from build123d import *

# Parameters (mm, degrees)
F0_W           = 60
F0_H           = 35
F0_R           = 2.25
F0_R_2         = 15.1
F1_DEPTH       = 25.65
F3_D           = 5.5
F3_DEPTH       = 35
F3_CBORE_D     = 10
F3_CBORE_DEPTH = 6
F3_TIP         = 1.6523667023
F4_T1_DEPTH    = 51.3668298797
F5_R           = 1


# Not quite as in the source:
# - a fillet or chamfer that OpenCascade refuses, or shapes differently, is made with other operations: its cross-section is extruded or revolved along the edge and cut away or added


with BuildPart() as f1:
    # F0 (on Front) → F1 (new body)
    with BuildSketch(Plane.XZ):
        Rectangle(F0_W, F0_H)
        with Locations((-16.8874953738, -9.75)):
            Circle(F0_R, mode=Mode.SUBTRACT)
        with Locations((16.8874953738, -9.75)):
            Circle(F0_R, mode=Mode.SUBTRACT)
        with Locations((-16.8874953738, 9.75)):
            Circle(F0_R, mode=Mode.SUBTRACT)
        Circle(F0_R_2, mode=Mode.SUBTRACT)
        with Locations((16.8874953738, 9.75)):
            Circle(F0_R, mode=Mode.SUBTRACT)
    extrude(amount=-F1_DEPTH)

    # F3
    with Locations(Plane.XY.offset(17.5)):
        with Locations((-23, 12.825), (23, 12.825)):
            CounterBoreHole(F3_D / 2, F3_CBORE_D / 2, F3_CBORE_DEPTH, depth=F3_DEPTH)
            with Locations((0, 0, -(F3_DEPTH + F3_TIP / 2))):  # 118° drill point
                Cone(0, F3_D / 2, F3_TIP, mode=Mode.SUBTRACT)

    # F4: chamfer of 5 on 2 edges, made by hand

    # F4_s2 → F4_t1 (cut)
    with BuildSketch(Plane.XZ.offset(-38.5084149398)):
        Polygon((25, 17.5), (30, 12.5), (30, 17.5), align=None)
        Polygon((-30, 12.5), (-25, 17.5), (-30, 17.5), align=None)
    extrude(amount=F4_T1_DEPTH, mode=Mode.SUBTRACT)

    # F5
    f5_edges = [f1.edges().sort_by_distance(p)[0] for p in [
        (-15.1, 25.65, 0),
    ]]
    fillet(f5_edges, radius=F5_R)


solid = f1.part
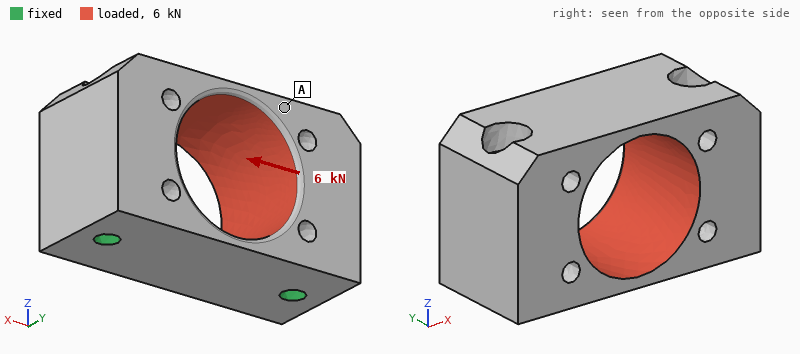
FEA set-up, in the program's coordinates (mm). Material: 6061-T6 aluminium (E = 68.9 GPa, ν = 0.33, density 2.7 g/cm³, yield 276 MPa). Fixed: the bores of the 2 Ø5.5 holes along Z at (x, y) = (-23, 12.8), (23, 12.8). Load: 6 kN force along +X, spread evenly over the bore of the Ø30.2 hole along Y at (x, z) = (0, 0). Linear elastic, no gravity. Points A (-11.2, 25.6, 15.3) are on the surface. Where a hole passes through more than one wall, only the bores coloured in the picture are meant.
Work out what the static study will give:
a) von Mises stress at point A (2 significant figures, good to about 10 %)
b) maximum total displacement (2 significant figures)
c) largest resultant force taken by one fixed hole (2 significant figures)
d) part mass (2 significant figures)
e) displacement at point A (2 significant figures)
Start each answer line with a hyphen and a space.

- 4.1 MPa
- 4.7 µm
- 3.0 kN
- 84 g
- 3.9 µm
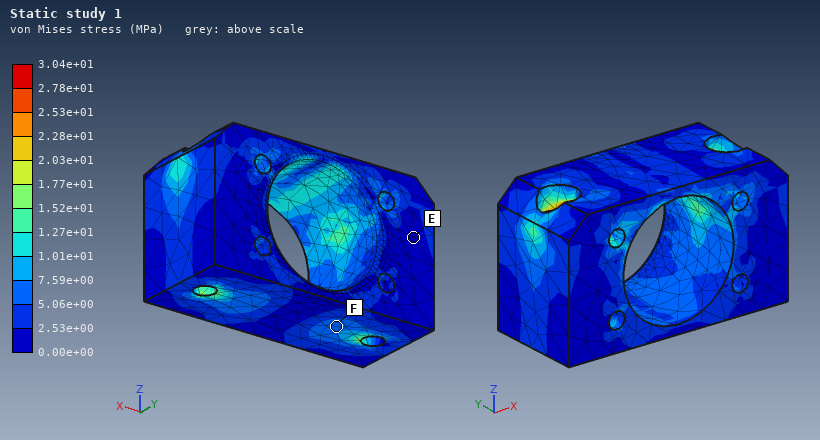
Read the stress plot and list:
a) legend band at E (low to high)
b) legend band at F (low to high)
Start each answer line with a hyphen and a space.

- 0.00e+00 to 2.53e+00 MPa
- 5.06e+00 to 7.59e+00 MPa
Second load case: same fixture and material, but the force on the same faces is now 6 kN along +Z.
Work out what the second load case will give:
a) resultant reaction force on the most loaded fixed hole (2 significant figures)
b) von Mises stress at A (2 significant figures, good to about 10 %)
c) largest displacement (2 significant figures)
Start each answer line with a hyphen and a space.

- 3.0 kN
- 3.5 MPa
- 12 µm
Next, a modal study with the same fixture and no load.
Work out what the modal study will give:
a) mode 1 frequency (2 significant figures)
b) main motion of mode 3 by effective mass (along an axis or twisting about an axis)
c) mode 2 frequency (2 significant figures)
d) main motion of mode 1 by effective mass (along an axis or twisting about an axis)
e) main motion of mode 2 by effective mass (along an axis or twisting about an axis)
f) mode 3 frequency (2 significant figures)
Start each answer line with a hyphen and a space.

- 21 kHz
- twisting about X
- 25 kHz
- along Y
- along X
- 27 kHz
